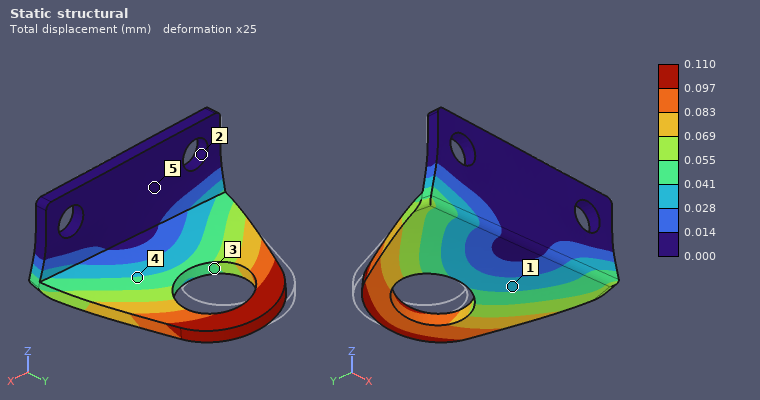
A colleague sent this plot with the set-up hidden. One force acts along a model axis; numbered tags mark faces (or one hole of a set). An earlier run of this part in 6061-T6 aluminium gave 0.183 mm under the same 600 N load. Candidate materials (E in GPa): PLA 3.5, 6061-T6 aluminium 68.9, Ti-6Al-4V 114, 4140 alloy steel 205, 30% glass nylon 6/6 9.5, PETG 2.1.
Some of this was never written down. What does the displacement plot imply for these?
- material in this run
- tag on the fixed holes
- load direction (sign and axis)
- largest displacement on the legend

Ti-6Al-4V
2
+X
0.110 mm
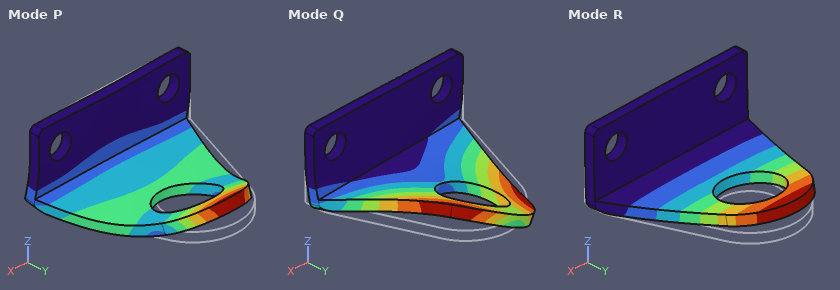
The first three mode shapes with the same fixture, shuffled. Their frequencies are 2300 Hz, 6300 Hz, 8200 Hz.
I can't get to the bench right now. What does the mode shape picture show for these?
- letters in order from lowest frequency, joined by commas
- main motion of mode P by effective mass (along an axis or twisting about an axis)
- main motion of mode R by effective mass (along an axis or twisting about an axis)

R, Q, P
along Y
along Z
